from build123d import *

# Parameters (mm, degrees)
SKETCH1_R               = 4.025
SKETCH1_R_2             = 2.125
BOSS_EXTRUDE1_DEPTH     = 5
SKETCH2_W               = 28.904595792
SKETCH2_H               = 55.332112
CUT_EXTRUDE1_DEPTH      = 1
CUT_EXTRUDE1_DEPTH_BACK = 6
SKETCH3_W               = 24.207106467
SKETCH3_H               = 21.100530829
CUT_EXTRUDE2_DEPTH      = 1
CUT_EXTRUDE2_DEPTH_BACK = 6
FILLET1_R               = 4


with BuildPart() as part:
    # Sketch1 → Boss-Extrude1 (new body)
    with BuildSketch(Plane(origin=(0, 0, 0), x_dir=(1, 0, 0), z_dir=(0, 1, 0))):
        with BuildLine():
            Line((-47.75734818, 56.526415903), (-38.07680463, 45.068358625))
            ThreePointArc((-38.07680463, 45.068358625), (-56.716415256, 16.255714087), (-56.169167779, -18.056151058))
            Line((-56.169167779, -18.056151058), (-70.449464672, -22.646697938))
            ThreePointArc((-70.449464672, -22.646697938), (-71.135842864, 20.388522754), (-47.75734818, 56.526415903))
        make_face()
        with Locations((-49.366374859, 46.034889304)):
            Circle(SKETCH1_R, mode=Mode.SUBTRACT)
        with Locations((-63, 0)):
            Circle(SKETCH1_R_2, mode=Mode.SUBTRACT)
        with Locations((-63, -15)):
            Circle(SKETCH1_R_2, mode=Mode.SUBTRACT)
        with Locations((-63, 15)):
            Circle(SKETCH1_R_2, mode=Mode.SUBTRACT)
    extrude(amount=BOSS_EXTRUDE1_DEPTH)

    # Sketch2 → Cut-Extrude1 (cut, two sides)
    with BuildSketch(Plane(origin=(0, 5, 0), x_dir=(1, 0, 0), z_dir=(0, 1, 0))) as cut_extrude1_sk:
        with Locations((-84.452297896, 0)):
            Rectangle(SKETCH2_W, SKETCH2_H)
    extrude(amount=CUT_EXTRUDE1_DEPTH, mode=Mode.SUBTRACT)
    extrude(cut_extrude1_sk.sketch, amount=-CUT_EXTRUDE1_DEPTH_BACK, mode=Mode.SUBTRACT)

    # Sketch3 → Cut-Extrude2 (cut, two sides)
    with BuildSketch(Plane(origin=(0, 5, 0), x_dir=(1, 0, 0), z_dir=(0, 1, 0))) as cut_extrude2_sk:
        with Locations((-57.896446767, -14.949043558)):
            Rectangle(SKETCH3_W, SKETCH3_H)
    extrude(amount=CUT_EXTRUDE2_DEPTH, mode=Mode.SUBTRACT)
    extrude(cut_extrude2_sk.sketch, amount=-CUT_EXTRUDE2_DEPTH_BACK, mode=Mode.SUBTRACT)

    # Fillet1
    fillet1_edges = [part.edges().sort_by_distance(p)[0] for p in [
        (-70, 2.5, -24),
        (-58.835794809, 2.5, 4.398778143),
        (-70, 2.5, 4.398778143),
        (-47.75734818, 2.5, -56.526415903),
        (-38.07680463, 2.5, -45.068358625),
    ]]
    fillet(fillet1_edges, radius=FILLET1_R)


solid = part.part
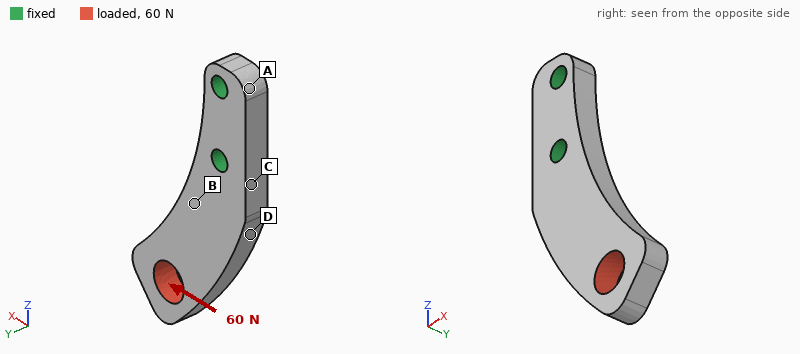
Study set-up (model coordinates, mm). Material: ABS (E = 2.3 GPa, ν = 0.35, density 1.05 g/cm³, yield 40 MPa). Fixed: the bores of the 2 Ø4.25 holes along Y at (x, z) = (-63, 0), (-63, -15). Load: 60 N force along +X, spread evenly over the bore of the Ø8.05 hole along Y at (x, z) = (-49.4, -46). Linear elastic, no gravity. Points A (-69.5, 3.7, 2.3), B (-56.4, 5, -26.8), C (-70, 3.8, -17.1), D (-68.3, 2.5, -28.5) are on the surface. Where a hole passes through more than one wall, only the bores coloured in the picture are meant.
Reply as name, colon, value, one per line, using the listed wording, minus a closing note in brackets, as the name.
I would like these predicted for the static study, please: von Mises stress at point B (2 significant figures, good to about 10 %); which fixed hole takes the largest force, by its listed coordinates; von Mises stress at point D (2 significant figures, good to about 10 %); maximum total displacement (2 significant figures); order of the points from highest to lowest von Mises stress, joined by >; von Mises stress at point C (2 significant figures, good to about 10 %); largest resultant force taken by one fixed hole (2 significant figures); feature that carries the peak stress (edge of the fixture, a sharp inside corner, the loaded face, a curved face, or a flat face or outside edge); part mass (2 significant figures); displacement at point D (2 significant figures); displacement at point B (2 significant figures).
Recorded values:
von Mises stress at point B: 3.1 MPa
which fixed hole takes the largest force, by its listed coordinates: (-63, -15)
von Mises stress at point D: 6.1 MPa
maximum total displacement: 0.56 mm
order of the points from highest to lowest von Mises stress, joined by >: C > D > B > A
von Mises stress at point C: 10 MPa
largest resultant force taken by one fixed hole: 120 N
feature that carries the peak stress: edge of the fixture
part mass: 4.0 g
displacement at point D: 0.13 mm
displacement at point B: 0.12 mm
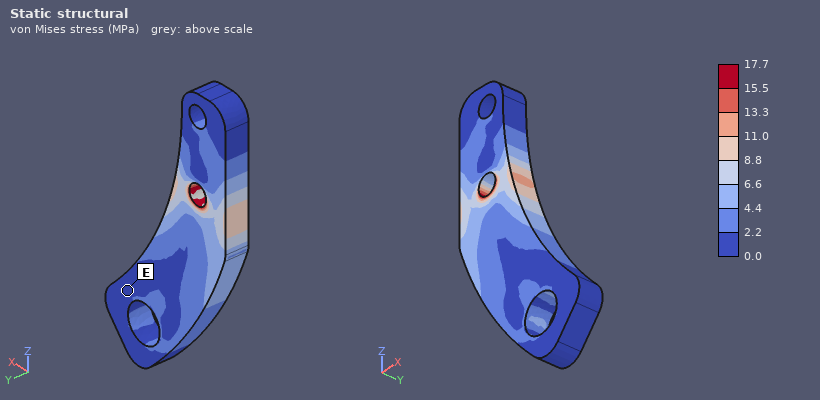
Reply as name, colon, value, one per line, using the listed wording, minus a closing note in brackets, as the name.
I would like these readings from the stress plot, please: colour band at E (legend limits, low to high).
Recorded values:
colour band at E: 0.0 to 2.2 MPa
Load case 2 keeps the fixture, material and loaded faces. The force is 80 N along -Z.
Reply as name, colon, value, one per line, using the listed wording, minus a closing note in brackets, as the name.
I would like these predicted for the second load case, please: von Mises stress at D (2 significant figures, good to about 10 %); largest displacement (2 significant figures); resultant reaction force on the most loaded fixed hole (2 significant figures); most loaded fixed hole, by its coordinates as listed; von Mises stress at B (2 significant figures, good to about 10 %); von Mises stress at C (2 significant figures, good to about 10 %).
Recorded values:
von Mises stress at D: 3.7 MPa
largest displacement: 0.37 mm
resultant reaction force on the most loaded fixed hole: 93 N
most loaded fixed hole, by its coordinates as listed: (-63, -15)
von Mises stress at B: 3.4 MPa
von Mises stress at C: 5.7 MPa
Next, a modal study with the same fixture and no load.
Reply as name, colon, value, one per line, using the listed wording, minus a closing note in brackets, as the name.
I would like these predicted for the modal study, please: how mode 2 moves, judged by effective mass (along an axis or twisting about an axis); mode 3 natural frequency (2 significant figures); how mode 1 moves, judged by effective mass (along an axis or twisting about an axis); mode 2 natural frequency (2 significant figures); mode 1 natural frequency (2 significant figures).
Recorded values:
how mode 2 moves, judged by effective mass: along X
mode 3 natural frequency: 2900 Hz
how mode 1 moves, judged by effective mass: along Y
mode 2 natural frequency: 1600 Hz
mode 1 natural frequency: 780 Hz
